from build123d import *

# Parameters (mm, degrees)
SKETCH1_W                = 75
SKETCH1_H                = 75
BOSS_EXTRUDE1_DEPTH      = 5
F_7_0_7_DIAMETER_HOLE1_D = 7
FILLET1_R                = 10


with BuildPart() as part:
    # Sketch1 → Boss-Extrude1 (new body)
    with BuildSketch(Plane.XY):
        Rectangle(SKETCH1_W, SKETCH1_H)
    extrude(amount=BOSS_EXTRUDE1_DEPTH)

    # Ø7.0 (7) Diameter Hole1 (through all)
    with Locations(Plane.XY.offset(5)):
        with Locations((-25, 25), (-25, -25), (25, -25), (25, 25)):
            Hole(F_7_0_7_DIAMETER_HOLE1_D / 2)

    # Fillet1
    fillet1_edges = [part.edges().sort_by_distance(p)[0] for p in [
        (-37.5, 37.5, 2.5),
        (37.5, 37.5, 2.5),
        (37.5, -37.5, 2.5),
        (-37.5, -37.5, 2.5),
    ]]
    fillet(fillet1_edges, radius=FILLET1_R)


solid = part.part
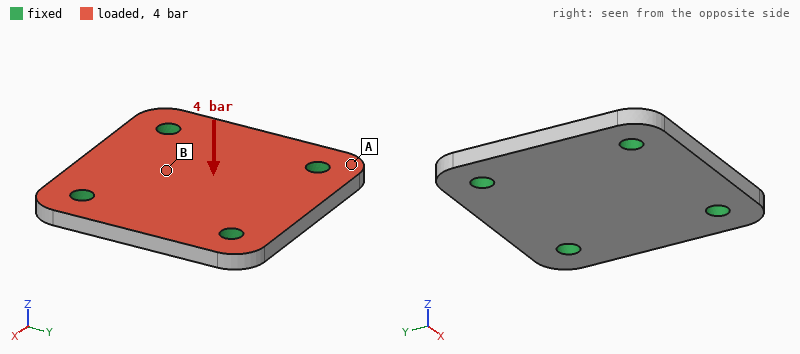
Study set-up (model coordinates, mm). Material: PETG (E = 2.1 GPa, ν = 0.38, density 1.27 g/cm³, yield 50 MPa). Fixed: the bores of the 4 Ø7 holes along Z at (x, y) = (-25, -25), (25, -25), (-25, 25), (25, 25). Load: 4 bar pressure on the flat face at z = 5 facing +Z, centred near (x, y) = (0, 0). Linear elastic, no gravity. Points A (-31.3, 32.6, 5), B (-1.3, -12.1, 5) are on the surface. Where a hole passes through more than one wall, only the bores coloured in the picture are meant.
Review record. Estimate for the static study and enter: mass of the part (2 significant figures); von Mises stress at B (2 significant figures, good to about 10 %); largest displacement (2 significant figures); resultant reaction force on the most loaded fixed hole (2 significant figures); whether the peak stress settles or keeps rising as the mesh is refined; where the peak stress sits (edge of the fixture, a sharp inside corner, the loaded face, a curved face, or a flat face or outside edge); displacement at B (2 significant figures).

34 g
8.6 MPa
0.54 mm
540 N
keeps rising
edge of the fixture
0.46 mm
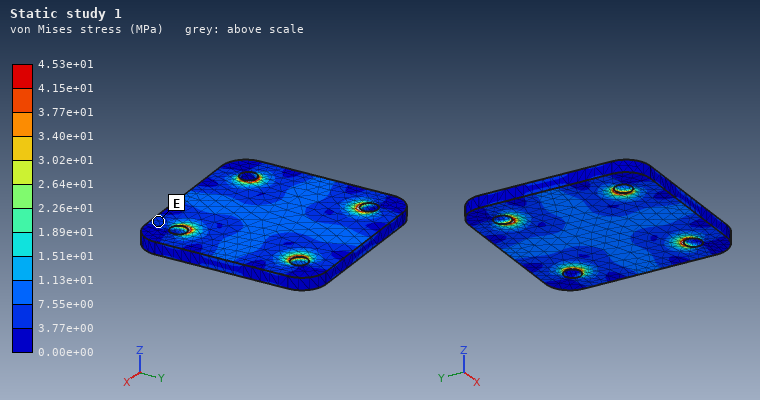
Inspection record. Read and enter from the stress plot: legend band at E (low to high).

3.77e+00 to 7.55e+00 MPa
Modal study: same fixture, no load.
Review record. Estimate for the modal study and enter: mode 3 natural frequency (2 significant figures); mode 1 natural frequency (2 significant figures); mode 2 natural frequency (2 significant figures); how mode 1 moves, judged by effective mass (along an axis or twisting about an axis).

2900 Hz
2100 Hz
2800 Hz
along Z
